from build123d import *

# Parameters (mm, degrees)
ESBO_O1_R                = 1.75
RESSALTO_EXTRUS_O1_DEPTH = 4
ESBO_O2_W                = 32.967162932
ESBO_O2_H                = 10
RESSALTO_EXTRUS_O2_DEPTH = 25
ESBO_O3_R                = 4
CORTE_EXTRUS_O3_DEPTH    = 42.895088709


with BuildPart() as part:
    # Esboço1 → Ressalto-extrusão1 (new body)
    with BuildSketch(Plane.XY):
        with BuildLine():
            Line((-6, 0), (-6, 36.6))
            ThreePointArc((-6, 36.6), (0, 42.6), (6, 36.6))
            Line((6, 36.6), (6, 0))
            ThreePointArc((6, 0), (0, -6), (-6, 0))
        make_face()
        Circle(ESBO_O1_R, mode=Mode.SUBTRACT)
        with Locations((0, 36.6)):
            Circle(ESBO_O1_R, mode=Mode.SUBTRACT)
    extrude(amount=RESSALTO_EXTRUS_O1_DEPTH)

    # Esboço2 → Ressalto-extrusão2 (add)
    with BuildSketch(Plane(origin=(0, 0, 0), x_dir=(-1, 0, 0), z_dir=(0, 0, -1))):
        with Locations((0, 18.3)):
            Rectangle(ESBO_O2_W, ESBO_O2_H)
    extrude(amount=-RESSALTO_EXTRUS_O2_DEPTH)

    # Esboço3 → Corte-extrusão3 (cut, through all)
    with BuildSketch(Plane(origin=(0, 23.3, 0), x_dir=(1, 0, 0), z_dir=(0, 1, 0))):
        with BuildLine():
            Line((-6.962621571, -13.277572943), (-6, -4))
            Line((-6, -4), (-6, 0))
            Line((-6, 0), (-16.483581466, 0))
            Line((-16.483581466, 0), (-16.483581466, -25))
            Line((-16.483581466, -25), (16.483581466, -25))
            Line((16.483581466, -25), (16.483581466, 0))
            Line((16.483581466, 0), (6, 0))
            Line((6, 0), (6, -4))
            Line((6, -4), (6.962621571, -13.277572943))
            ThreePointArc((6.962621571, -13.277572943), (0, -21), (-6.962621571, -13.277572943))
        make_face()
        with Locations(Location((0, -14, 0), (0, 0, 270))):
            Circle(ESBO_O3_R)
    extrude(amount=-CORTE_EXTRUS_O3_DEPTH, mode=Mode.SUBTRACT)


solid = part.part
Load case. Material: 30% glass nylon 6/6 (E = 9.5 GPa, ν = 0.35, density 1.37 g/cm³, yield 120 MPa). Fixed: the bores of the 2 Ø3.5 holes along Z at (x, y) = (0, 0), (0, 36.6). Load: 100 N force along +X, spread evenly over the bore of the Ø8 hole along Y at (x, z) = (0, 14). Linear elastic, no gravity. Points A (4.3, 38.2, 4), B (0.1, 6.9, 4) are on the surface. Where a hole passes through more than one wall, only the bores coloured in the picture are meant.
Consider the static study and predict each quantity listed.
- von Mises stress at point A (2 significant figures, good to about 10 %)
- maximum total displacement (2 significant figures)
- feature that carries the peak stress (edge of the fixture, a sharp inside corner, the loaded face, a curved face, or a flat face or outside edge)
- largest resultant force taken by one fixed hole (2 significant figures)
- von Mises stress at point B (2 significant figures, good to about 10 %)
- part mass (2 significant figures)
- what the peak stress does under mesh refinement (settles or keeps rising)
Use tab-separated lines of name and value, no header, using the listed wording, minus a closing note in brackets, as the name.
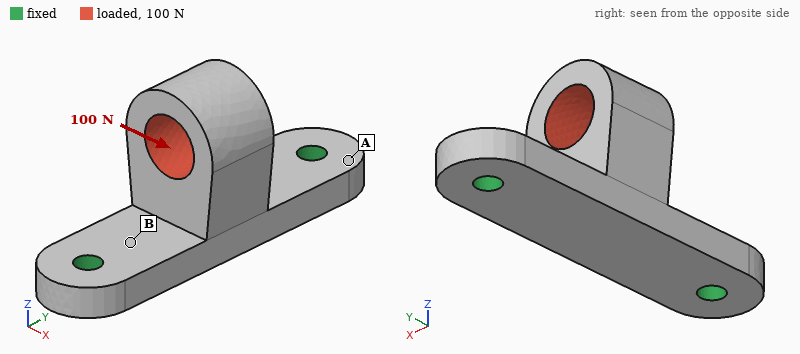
von Mises stress at point A	4.5 MPa
maximum total displacement	0.22 mm
feature that carries the peak stress	edge of the fixture
largest resultant force taken by one fixed hole	50 N
von Mises stress at point B	20 MPa
part mass	5.1 g
what the peak stress does under mesh refinement	keeps rising
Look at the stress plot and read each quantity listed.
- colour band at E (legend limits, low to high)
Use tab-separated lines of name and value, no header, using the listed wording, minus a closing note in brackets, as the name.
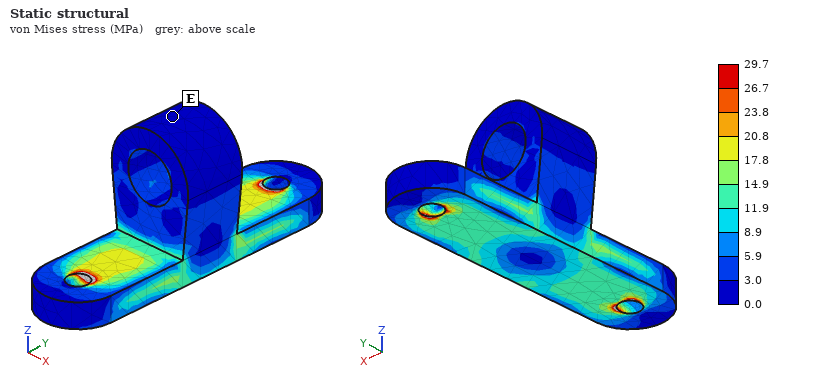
colour band at E	0.0 to 3.0 MPa
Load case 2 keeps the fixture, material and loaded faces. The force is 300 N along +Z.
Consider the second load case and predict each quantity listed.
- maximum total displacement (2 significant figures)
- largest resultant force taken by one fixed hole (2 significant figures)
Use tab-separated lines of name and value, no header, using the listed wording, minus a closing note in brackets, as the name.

maximum total displacement	87 µm
largest resultant force taken by one fixed hole	160 N
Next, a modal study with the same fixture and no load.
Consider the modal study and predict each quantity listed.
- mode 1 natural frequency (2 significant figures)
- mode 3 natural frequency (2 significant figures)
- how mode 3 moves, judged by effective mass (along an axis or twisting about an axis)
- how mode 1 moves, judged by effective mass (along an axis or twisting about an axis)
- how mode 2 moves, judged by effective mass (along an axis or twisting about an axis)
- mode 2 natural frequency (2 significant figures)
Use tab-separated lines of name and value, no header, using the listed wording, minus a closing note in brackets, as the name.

mode 1 natural frequency	3000 Hz
mode 3 natural frequency	6100 Hz
how mode 3 moves, judged by effective mass	along Y
how mode 1 moves, judged by effective mass	along X
how mode 2 moves, judged by effective mass	along Z
mode 2 natural frequency	5400 Hz
